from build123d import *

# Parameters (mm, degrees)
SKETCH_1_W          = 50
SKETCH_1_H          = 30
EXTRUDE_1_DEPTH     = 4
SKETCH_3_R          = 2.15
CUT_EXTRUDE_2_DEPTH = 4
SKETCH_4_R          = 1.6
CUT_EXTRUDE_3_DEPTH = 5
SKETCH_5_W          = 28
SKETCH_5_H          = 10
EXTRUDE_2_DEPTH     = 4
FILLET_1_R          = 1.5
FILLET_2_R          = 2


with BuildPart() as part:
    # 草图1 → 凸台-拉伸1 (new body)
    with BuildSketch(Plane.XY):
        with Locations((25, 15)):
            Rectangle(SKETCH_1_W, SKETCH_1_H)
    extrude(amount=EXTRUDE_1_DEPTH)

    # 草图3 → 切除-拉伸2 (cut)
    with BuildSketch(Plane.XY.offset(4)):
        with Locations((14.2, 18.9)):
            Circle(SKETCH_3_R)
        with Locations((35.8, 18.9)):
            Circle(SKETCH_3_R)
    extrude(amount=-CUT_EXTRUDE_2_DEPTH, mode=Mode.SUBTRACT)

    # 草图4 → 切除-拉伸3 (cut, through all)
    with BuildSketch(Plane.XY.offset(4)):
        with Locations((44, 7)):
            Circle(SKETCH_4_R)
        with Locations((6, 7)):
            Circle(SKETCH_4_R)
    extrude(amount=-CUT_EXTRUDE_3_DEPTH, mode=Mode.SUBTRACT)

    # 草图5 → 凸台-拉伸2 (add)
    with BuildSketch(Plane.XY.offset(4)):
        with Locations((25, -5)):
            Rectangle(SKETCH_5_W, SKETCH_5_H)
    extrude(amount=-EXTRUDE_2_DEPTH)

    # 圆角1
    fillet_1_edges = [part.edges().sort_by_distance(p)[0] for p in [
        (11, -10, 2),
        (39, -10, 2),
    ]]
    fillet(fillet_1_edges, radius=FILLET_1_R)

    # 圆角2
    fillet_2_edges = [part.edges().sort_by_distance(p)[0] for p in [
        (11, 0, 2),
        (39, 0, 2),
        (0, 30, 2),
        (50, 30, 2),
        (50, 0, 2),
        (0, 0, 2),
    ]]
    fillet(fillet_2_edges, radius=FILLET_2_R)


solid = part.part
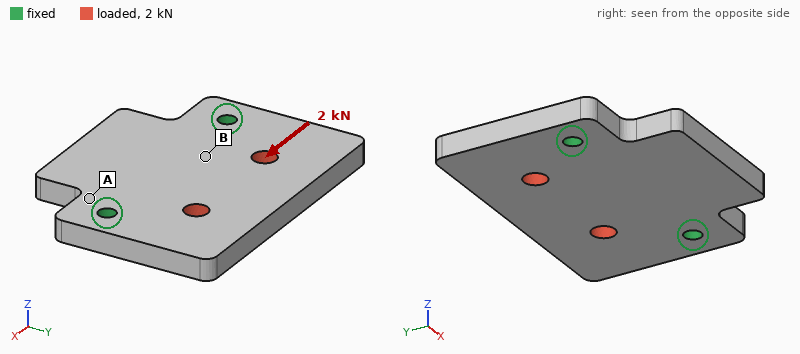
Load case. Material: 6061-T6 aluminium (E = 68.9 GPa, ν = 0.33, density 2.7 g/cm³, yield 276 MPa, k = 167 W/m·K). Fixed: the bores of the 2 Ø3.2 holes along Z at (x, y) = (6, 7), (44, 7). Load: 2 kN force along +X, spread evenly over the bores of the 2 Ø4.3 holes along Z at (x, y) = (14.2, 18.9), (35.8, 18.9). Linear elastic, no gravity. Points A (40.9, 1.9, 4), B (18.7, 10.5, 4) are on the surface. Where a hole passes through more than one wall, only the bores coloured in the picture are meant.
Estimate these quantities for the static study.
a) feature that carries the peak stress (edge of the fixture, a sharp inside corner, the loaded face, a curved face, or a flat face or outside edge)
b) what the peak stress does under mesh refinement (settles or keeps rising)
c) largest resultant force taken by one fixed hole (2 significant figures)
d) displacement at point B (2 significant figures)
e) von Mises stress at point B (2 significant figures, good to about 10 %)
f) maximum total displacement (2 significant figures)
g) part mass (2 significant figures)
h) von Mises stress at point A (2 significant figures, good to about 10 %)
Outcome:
edge of the fixture
keeps rising
1.2 kN
3.5 µm
16 MPa
9.4 µm
19 g
7.2 MPa
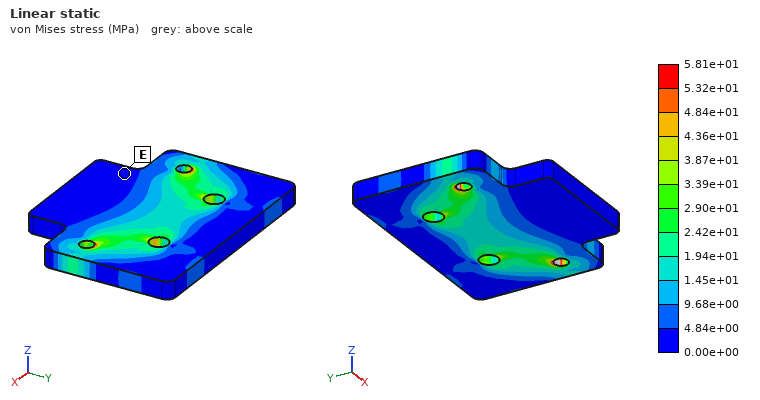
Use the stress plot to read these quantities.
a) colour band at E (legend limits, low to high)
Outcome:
0.00e+00 to 4.84e+00 MPa
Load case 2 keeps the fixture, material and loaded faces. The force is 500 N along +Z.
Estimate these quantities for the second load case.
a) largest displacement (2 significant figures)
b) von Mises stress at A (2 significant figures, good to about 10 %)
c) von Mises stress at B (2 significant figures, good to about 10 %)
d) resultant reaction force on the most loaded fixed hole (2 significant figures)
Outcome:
78 µm
23 MPa
19 MPa
250 N
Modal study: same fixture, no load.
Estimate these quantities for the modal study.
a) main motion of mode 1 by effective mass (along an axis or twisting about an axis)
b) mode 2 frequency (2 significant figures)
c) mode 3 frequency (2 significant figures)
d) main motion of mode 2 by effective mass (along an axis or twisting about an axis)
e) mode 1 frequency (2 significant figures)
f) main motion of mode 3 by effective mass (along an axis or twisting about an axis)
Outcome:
along Z
7900 Hz
8600 Hz
along Z
4700 Hz
twisting about Y
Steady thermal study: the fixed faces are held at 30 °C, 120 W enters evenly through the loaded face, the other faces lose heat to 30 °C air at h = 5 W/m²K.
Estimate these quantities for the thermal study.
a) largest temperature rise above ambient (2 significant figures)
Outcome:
83 K
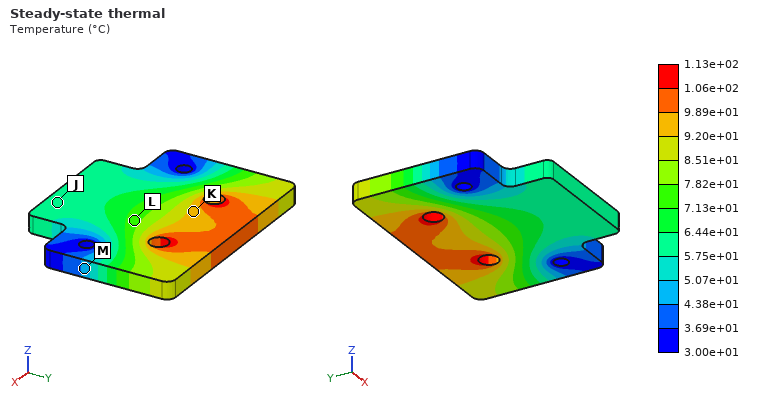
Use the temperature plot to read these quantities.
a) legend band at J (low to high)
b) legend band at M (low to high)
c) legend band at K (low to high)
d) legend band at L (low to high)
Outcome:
5.75e+01 to 6.44e+01 °C
4.38e+01 to 5.07e+01 °C
9.20e+01 to 9.89e+01 °C
7.13e+01 to 7.82e+01 °C
